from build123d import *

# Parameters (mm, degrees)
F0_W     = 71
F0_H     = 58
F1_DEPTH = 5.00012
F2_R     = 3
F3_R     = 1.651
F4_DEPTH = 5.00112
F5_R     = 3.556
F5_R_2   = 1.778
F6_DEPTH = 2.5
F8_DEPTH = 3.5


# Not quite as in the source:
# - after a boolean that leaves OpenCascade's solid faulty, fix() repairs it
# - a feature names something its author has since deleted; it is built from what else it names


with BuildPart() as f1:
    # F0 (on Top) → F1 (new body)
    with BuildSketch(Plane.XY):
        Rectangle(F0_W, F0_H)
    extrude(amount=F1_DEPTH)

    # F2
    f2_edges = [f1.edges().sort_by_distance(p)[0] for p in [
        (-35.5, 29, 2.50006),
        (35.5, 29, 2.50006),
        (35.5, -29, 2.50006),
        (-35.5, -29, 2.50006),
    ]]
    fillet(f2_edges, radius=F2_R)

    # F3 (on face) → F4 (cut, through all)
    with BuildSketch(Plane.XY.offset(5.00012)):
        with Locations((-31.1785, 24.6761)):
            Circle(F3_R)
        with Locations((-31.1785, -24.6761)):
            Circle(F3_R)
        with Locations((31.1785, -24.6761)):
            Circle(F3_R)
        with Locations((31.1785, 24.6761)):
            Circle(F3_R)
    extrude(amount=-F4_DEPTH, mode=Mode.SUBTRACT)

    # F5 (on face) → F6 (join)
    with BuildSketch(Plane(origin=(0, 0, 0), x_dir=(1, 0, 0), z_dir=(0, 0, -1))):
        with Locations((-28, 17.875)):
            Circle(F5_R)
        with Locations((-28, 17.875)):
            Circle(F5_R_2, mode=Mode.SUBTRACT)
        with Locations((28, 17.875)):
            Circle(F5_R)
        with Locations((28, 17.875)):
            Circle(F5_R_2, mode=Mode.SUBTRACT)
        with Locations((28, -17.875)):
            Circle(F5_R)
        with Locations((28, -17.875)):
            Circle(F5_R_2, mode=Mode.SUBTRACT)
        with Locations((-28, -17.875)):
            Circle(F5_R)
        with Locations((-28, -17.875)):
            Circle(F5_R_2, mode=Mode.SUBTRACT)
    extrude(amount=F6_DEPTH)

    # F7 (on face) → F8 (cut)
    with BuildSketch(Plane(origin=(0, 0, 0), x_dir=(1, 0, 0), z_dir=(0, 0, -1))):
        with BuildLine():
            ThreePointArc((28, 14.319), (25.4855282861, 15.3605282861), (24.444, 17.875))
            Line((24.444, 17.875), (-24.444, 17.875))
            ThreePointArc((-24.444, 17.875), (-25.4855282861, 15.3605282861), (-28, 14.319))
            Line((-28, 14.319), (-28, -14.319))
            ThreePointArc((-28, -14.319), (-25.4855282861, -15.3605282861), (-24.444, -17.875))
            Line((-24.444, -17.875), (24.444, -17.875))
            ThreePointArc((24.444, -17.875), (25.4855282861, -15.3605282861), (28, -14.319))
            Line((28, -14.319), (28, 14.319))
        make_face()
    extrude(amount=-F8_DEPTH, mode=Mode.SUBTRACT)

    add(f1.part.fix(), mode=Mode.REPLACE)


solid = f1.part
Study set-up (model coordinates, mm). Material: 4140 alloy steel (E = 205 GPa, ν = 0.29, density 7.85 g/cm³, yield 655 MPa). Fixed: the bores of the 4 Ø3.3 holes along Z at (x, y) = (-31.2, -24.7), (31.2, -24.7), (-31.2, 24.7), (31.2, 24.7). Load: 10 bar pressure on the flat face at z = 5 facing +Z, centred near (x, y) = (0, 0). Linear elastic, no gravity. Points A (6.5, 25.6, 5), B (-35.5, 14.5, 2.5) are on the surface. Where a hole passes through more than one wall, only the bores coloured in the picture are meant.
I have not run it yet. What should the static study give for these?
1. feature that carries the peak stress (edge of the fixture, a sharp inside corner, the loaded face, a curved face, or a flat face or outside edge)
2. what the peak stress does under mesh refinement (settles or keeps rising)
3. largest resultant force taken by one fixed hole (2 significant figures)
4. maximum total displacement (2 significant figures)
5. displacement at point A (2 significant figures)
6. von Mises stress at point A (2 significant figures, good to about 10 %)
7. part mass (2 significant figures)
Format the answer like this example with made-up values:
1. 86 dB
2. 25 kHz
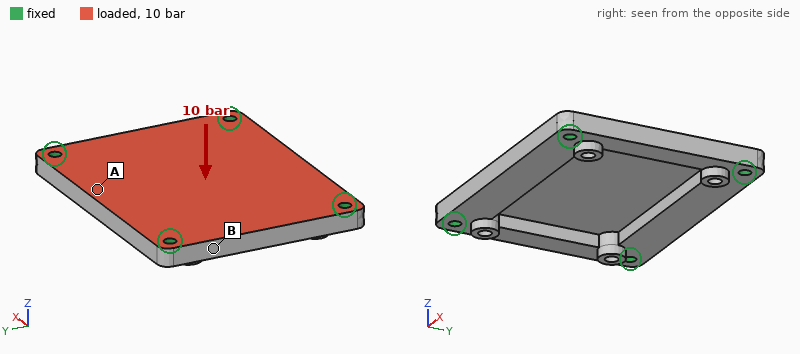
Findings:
1. edge of the fixture
2. keeps rising
3. 1.3 kN
4. 0.13 mm
5. 0.033 mm
6. 57 MPa
7. 110 g
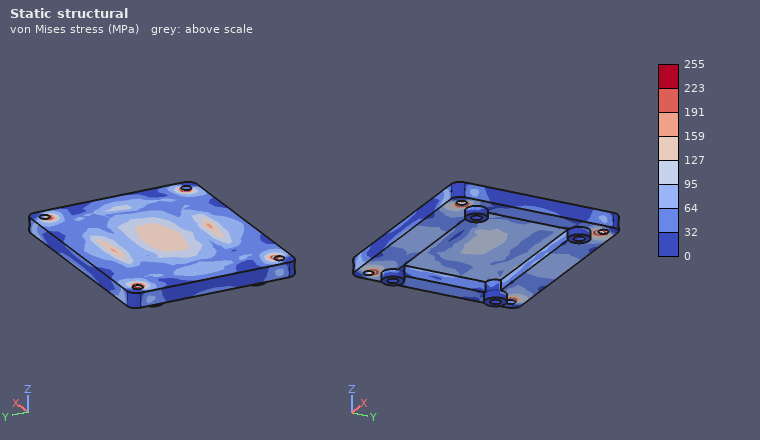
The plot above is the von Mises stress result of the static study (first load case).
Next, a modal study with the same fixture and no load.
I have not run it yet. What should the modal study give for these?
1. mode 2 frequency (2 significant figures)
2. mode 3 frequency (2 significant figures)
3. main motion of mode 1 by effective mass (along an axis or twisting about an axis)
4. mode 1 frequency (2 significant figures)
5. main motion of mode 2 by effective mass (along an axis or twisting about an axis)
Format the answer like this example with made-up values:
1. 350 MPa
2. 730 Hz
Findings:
1. 6500 Hz
2. 8100 Hz
3. along Z
4. 4900 Hz
5. twisting about X
